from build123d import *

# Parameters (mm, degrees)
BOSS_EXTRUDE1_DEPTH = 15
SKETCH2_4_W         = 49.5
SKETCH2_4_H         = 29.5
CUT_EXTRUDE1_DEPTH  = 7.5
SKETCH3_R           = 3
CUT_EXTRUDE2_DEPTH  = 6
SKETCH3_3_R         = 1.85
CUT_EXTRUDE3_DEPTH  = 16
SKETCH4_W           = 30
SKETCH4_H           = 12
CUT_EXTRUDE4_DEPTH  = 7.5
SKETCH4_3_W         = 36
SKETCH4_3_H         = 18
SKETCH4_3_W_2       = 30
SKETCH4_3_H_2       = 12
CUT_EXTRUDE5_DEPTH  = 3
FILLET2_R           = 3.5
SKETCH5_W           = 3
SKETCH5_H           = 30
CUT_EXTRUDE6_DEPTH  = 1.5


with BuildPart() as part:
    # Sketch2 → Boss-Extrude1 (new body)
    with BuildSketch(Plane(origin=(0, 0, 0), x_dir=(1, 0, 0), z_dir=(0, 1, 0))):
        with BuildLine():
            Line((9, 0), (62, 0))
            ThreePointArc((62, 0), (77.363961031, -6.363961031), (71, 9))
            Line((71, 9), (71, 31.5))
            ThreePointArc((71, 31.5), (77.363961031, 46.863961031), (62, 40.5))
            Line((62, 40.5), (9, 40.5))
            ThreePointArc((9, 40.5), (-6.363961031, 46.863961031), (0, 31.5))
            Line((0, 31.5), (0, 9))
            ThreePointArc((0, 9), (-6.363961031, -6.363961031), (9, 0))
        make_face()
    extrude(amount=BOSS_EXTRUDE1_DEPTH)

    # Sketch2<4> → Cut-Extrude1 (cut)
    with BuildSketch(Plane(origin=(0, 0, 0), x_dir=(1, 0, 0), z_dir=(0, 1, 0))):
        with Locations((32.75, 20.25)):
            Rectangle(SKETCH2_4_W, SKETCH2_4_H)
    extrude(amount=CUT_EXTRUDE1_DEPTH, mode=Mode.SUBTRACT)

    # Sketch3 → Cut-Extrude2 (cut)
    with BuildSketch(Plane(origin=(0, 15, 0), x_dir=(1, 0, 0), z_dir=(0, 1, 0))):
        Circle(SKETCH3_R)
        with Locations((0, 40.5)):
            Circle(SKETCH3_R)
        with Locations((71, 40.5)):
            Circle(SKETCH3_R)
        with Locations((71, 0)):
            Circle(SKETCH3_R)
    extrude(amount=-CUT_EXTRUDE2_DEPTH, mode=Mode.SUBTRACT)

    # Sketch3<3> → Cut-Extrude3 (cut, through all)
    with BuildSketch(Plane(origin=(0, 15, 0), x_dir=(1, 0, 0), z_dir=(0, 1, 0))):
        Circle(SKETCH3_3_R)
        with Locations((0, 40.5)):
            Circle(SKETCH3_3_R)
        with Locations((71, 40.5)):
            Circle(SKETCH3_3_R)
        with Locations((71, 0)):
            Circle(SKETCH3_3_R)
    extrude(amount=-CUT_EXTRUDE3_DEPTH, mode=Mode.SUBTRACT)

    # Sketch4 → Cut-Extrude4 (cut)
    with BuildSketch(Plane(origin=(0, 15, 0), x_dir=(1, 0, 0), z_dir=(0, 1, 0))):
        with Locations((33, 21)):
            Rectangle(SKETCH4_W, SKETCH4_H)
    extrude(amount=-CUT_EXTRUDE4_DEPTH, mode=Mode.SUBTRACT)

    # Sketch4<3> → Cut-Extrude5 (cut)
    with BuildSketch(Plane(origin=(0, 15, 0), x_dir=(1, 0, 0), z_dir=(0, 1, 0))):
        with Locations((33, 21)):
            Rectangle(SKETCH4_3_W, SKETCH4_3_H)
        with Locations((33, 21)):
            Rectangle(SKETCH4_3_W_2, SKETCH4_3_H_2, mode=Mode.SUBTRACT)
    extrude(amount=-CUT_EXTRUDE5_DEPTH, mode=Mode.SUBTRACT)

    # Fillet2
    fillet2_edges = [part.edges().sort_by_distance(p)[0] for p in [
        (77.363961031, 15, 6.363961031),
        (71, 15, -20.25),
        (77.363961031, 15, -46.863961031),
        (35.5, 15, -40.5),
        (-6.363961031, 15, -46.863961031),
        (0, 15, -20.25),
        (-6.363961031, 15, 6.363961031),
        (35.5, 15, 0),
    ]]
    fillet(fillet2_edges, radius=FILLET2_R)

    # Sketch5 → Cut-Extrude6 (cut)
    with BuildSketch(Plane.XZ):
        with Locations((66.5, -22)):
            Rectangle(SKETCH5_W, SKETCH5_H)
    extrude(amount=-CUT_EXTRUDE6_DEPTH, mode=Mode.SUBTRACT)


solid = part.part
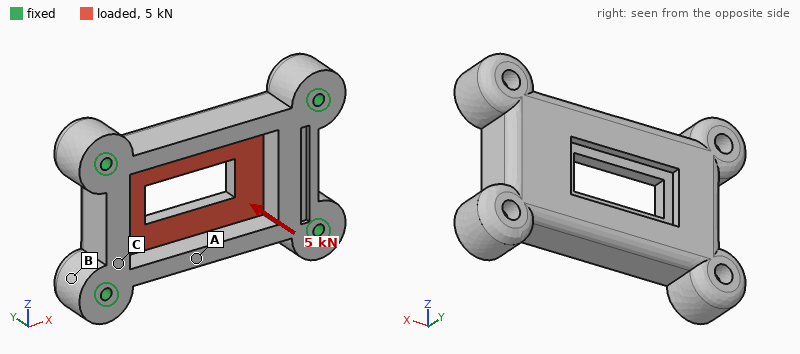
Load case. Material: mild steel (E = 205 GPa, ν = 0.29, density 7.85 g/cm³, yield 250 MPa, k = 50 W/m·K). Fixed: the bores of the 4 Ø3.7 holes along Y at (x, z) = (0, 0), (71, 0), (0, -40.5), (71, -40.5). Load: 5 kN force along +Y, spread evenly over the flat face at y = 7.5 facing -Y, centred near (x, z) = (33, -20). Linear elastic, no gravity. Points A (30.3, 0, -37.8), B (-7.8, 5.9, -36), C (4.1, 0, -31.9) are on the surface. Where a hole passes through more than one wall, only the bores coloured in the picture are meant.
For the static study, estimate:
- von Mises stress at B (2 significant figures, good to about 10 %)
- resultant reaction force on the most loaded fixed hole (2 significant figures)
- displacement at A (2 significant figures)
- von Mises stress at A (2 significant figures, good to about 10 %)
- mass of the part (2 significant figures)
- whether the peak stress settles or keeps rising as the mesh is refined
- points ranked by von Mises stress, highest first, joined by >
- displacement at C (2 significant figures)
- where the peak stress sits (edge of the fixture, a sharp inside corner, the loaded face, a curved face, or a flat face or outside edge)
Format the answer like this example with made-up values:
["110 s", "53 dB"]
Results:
["8.4 MPa", "1.8 kN", "11 µm", "30 MPa", "300 g", "keeps rising", "A > C > B", "3.1 µm", "edge of the fixture"]
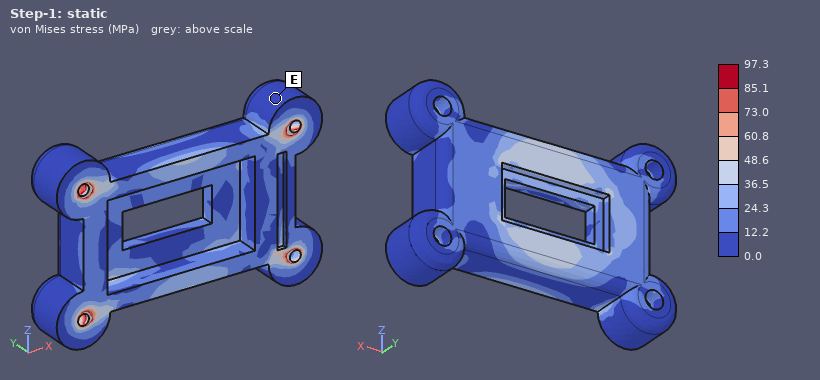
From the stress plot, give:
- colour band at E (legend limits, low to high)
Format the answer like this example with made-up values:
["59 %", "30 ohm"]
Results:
["0.0 to 12.2 MPa"]
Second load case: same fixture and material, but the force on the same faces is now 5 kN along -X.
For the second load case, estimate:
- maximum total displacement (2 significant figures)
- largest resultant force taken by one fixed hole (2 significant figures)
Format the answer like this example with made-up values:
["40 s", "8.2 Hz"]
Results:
["2.2 µm", "1.4 kN"]
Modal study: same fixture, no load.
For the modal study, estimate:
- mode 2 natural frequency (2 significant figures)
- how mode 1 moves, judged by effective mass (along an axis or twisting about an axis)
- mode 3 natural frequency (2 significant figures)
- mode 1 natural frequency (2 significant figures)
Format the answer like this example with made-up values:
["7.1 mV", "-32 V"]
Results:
["12 kHz", "along Y", "17 kHz", "9700 Hz"]
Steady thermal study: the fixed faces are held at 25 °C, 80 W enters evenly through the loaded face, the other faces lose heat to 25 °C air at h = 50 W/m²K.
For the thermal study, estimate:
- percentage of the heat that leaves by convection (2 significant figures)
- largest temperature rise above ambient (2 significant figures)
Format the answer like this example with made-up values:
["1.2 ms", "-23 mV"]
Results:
["17 %", "57 K"]
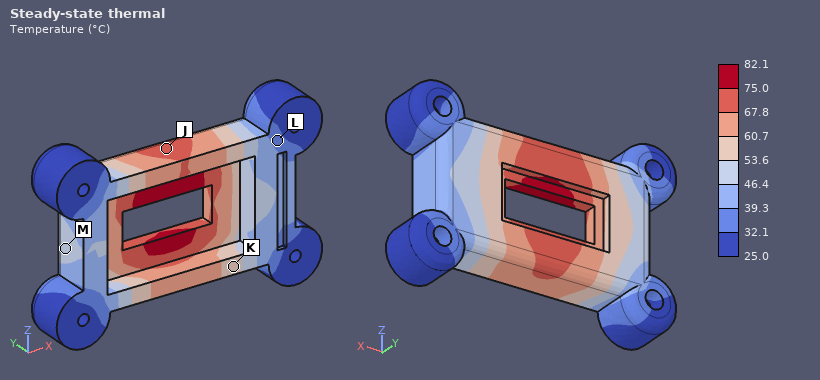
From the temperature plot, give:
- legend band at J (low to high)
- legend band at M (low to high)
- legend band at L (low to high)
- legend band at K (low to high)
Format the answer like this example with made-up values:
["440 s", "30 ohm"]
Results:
["67.8 to 75.0 °C", "46.4 to 53.6 °C", "32.1 to 39.3 °C", "53.6 to 60.7 °C"]
